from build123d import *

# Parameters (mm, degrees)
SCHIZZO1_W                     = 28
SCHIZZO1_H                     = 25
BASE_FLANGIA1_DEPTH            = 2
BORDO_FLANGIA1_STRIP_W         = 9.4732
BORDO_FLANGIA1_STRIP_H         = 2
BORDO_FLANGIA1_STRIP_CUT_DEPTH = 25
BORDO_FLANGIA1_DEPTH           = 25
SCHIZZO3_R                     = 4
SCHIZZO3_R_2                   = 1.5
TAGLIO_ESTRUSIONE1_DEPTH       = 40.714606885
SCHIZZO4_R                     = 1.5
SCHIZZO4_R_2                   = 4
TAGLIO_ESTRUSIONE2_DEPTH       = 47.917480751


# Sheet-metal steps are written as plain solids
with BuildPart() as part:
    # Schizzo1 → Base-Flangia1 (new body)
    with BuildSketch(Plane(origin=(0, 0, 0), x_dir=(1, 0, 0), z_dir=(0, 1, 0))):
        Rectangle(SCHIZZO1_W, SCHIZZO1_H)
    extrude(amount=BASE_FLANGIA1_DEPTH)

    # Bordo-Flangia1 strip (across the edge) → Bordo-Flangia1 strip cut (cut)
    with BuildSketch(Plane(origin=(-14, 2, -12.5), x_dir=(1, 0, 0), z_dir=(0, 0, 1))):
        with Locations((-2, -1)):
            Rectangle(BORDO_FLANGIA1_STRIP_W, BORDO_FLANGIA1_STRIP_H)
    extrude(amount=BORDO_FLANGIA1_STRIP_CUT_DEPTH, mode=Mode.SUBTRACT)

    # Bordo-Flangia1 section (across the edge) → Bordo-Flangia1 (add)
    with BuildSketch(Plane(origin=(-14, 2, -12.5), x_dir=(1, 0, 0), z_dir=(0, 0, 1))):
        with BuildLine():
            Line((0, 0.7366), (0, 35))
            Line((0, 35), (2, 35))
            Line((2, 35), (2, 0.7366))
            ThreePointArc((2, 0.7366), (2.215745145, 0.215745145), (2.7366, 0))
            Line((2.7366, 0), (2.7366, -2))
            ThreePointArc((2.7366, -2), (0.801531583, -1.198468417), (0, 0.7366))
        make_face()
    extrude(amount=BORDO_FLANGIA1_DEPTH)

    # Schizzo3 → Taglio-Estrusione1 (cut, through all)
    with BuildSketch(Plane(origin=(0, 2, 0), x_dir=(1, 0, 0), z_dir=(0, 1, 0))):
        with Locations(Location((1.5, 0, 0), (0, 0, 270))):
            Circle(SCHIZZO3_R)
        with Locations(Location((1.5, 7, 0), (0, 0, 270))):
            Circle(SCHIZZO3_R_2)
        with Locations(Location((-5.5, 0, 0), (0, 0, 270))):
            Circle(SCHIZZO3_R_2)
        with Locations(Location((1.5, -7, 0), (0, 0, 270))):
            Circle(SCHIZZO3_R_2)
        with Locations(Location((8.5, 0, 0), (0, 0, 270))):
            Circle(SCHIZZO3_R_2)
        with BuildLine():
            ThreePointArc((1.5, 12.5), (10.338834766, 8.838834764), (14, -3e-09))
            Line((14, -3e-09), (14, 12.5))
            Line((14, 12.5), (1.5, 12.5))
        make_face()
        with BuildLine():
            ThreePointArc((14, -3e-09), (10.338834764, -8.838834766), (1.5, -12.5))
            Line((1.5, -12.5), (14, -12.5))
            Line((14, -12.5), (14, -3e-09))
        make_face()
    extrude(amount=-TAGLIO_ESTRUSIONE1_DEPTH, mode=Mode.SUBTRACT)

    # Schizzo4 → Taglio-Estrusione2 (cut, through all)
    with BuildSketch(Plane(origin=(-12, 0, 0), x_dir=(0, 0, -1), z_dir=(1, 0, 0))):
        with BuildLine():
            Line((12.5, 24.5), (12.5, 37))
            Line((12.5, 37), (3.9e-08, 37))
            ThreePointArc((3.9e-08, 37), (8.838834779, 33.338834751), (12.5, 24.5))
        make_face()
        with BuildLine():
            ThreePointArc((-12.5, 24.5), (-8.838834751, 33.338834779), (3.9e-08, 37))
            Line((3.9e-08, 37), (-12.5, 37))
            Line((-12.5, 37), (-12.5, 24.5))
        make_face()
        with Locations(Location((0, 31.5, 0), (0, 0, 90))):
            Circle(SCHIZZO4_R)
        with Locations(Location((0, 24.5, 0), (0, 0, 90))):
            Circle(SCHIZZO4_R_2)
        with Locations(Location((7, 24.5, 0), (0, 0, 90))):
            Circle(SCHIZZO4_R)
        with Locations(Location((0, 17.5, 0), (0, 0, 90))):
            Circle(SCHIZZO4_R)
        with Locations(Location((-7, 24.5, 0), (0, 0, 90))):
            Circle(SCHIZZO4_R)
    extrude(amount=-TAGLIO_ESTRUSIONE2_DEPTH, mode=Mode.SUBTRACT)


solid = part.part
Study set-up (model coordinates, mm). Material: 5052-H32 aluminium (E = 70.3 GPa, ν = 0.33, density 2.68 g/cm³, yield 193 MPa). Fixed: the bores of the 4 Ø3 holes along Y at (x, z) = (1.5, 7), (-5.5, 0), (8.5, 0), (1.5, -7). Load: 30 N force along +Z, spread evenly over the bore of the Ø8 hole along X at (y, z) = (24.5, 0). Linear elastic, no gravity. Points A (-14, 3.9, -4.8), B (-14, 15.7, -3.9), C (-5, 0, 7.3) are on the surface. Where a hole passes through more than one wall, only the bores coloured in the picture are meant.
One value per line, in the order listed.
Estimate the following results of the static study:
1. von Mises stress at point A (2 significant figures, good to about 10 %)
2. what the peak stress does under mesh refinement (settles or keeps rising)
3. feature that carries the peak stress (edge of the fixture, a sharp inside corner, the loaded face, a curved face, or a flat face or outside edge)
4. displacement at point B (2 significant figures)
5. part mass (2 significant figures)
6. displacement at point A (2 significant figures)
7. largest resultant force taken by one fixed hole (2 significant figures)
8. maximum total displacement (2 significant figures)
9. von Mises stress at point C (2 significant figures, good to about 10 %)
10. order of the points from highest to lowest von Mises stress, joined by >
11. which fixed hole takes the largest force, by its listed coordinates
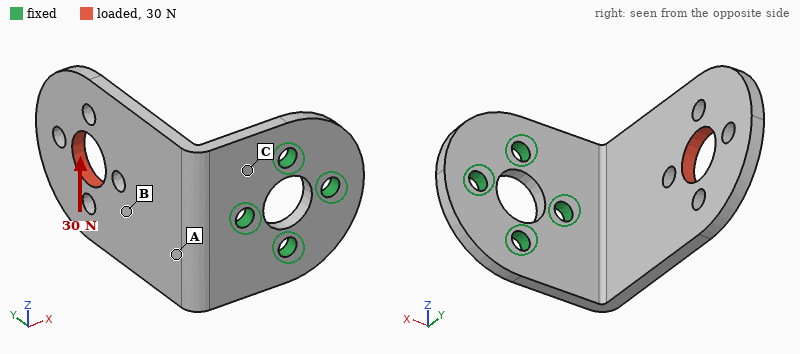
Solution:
11 MPa
keeps rising
edge of the fixture
32 µm
6.8 g
12 µm
28 N
79 µm
18 MPa
C > A > B
(-5.5, 0)
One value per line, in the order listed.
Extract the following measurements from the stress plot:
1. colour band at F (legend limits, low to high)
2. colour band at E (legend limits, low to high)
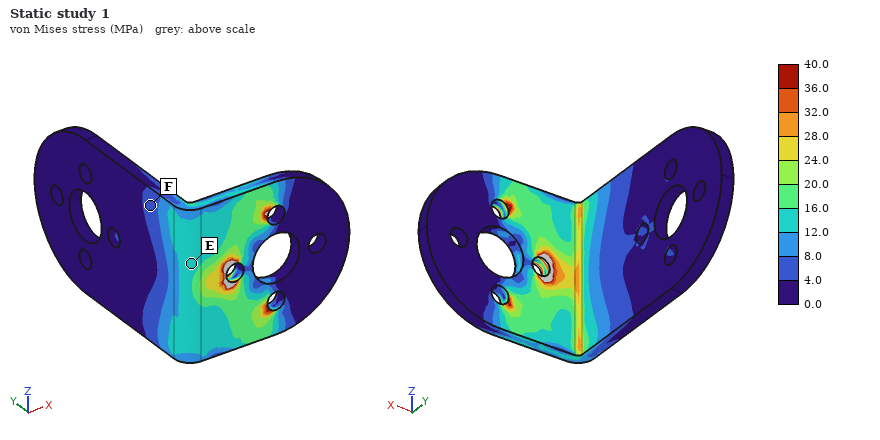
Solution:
4.0 to 8.0 MPa
12.0 to 16.0 MPa
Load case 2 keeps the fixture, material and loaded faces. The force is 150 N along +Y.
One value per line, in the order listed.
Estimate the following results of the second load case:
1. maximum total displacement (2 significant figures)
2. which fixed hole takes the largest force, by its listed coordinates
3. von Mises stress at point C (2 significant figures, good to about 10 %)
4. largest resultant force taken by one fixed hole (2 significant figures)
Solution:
0.14 mm
(-5.5, 0)
23 MPa
190 N
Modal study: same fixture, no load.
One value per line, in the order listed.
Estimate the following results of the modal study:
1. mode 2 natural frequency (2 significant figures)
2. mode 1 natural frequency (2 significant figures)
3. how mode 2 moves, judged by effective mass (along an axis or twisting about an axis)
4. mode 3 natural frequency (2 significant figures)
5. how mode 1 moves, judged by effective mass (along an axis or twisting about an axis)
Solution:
2200 Hz
1200 Hz
along Z
4500 Hz
along X
